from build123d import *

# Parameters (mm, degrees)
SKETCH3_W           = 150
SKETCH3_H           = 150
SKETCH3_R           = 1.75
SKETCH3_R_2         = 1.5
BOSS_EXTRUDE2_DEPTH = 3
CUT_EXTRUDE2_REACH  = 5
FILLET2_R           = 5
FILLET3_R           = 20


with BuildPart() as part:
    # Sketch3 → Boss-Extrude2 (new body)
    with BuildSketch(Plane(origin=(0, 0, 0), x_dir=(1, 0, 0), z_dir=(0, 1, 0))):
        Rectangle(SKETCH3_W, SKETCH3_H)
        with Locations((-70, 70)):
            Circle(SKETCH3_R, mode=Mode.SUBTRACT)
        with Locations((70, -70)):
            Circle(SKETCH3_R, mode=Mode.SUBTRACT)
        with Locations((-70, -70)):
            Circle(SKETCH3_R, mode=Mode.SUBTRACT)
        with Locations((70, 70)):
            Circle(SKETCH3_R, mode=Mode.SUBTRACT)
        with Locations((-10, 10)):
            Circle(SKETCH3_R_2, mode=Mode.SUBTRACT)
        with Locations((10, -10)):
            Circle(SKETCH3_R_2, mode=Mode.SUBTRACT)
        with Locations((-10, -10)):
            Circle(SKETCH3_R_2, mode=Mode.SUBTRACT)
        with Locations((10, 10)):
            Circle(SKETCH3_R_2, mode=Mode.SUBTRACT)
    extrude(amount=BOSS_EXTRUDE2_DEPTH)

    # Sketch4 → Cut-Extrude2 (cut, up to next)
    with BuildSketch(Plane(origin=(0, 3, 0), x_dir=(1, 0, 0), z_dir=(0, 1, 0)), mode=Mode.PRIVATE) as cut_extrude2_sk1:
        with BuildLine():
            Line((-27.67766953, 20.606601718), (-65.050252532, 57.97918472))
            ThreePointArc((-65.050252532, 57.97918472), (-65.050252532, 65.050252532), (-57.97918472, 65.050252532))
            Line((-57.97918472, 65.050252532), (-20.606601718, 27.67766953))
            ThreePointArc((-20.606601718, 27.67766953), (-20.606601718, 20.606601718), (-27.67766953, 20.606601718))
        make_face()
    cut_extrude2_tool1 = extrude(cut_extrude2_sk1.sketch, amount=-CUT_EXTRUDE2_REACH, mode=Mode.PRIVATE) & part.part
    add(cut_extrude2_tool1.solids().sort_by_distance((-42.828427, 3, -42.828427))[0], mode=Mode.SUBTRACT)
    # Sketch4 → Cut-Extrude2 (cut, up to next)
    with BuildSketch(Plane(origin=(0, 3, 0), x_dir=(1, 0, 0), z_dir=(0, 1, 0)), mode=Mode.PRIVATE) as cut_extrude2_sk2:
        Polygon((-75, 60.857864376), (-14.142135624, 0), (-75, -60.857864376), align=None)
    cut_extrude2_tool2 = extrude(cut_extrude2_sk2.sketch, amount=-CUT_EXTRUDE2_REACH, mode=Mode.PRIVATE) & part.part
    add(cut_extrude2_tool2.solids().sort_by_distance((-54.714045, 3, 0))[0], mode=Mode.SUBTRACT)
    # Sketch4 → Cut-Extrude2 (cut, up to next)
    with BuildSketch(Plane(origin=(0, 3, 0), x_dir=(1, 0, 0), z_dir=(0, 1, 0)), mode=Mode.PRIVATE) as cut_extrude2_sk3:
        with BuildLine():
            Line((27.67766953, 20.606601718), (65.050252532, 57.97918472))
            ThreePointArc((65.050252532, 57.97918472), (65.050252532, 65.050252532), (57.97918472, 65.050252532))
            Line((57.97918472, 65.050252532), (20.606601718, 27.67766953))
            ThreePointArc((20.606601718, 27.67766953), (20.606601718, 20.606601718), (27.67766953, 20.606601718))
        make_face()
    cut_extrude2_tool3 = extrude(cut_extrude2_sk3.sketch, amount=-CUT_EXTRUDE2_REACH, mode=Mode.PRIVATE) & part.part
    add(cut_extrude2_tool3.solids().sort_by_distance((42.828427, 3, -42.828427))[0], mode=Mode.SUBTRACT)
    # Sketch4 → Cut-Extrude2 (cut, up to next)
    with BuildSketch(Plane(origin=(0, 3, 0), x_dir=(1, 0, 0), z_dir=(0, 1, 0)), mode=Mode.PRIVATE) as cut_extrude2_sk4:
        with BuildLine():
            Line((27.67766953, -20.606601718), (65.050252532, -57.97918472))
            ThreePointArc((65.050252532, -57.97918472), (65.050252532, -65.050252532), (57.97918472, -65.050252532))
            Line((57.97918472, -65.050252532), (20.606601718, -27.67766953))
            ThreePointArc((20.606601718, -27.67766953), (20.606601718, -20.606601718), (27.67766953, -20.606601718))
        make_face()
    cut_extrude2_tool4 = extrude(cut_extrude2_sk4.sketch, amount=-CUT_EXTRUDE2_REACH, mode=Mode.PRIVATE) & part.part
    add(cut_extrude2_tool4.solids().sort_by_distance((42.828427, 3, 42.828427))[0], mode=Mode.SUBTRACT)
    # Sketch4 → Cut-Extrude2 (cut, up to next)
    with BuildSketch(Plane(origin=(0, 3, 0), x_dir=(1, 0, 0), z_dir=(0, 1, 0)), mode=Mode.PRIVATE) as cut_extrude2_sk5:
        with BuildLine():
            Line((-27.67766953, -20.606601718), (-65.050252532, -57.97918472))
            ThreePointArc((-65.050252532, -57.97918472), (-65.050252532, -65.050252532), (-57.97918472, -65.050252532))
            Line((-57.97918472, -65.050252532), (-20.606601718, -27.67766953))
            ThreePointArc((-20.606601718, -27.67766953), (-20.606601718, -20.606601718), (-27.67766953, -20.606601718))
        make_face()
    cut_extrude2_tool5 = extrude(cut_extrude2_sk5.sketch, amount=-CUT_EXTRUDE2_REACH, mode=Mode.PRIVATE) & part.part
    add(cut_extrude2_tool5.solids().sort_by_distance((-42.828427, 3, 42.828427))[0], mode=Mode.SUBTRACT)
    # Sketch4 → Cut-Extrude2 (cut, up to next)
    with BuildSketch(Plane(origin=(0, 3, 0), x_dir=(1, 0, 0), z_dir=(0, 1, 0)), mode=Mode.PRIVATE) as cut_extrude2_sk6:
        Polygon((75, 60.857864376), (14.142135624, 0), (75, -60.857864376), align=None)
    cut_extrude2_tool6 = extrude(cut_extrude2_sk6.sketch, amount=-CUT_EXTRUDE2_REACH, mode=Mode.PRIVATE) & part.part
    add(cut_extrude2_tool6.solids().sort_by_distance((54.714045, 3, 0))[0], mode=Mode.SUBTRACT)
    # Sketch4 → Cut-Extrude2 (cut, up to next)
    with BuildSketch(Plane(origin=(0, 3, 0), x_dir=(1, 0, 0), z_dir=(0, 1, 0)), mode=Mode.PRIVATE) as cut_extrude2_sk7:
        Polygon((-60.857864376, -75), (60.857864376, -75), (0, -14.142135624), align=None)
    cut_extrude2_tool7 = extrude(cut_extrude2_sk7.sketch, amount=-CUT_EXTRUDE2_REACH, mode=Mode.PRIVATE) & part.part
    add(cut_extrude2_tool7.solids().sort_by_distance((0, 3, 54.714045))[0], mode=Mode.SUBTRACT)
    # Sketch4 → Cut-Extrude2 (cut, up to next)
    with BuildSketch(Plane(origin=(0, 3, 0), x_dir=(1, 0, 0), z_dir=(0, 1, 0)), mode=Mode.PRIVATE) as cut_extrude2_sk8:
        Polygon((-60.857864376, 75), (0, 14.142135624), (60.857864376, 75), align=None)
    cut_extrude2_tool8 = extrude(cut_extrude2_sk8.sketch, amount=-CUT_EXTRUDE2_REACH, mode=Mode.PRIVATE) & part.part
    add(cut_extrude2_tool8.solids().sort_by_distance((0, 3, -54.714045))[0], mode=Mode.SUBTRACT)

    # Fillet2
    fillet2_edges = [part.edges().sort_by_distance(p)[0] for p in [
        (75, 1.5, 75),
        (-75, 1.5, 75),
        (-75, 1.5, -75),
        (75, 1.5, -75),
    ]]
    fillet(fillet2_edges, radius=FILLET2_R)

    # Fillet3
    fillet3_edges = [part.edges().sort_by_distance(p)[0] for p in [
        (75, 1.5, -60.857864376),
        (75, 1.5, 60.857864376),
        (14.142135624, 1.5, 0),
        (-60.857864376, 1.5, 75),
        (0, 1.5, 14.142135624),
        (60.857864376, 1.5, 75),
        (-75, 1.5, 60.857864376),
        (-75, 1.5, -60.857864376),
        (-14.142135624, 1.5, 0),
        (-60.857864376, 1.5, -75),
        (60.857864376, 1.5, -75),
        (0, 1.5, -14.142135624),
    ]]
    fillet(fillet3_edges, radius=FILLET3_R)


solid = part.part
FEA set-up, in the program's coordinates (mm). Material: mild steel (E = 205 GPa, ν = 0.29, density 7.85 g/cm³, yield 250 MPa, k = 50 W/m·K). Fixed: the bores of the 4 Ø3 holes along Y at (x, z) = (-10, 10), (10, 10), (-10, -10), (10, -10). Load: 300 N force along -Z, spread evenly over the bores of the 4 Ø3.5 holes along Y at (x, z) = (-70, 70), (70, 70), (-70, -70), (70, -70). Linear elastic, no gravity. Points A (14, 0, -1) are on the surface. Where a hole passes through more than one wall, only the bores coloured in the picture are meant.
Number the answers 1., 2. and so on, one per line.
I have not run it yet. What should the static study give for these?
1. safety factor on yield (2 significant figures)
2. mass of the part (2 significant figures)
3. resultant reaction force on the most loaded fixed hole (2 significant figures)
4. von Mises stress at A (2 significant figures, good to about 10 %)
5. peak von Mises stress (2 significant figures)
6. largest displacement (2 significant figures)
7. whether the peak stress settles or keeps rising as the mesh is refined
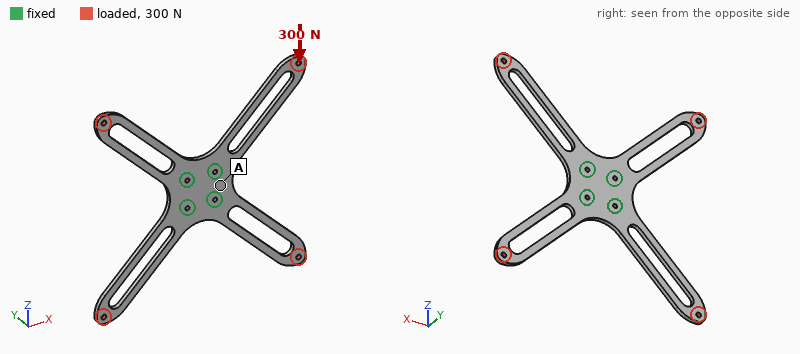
1. 3.4
2. 130 g
3. 78 N
4. 9.8 MPa
5. 73 MPa
6. 0.11 mm
7. settles
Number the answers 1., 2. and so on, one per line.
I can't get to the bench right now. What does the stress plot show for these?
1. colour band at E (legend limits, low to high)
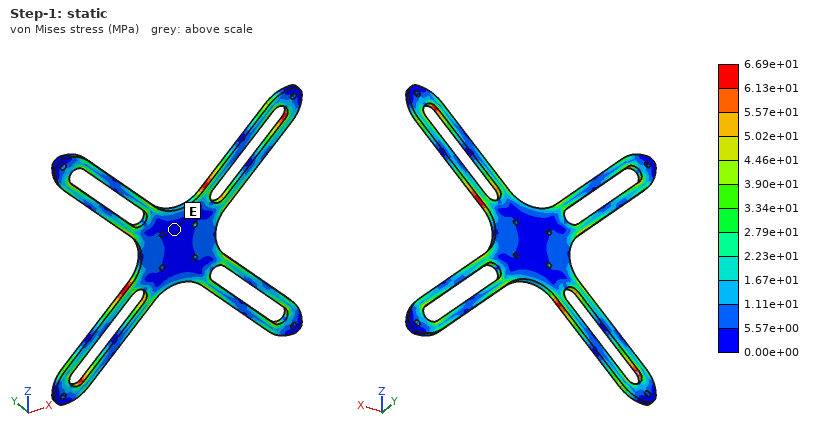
1. 0.00e+00 to 5.57e+00 MPa
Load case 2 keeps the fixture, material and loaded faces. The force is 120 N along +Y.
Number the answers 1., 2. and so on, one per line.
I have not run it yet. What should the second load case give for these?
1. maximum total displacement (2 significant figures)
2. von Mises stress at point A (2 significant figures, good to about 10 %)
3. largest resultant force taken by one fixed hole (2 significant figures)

1. 1.1 mm
2. 17 MPa
3. 30 N
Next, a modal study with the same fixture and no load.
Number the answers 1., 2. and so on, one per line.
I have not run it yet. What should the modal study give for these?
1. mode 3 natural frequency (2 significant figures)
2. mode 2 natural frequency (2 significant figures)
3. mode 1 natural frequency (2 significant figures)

1. 350 Hz
2. 350 Hz
3. 350 Hz
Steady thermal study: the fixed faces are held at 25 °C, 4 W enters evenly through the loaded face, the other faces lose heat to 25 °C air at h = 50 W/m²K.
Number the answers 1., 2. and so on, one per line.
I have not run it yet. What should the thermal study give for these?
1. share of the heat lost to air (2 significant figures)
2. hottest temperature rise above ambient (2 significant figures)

1. 88 %
2. 17 K
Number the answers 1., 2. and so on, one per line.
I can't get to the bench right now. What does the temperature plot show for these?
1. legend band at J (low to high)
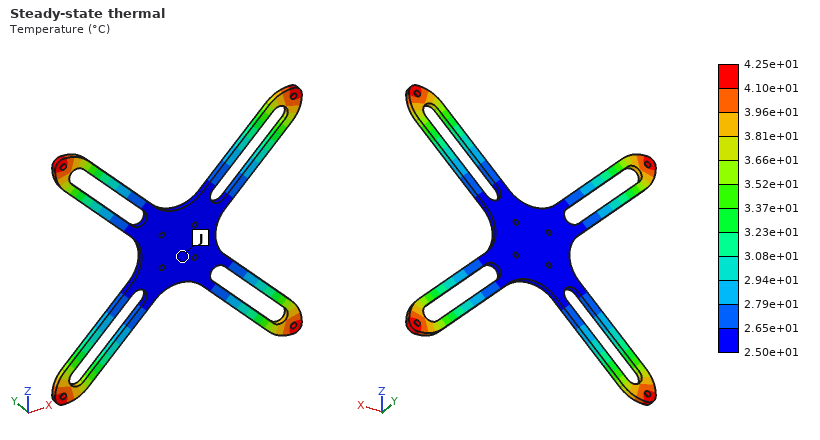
1. 2.50e+01 to 2.65e+01 °C
